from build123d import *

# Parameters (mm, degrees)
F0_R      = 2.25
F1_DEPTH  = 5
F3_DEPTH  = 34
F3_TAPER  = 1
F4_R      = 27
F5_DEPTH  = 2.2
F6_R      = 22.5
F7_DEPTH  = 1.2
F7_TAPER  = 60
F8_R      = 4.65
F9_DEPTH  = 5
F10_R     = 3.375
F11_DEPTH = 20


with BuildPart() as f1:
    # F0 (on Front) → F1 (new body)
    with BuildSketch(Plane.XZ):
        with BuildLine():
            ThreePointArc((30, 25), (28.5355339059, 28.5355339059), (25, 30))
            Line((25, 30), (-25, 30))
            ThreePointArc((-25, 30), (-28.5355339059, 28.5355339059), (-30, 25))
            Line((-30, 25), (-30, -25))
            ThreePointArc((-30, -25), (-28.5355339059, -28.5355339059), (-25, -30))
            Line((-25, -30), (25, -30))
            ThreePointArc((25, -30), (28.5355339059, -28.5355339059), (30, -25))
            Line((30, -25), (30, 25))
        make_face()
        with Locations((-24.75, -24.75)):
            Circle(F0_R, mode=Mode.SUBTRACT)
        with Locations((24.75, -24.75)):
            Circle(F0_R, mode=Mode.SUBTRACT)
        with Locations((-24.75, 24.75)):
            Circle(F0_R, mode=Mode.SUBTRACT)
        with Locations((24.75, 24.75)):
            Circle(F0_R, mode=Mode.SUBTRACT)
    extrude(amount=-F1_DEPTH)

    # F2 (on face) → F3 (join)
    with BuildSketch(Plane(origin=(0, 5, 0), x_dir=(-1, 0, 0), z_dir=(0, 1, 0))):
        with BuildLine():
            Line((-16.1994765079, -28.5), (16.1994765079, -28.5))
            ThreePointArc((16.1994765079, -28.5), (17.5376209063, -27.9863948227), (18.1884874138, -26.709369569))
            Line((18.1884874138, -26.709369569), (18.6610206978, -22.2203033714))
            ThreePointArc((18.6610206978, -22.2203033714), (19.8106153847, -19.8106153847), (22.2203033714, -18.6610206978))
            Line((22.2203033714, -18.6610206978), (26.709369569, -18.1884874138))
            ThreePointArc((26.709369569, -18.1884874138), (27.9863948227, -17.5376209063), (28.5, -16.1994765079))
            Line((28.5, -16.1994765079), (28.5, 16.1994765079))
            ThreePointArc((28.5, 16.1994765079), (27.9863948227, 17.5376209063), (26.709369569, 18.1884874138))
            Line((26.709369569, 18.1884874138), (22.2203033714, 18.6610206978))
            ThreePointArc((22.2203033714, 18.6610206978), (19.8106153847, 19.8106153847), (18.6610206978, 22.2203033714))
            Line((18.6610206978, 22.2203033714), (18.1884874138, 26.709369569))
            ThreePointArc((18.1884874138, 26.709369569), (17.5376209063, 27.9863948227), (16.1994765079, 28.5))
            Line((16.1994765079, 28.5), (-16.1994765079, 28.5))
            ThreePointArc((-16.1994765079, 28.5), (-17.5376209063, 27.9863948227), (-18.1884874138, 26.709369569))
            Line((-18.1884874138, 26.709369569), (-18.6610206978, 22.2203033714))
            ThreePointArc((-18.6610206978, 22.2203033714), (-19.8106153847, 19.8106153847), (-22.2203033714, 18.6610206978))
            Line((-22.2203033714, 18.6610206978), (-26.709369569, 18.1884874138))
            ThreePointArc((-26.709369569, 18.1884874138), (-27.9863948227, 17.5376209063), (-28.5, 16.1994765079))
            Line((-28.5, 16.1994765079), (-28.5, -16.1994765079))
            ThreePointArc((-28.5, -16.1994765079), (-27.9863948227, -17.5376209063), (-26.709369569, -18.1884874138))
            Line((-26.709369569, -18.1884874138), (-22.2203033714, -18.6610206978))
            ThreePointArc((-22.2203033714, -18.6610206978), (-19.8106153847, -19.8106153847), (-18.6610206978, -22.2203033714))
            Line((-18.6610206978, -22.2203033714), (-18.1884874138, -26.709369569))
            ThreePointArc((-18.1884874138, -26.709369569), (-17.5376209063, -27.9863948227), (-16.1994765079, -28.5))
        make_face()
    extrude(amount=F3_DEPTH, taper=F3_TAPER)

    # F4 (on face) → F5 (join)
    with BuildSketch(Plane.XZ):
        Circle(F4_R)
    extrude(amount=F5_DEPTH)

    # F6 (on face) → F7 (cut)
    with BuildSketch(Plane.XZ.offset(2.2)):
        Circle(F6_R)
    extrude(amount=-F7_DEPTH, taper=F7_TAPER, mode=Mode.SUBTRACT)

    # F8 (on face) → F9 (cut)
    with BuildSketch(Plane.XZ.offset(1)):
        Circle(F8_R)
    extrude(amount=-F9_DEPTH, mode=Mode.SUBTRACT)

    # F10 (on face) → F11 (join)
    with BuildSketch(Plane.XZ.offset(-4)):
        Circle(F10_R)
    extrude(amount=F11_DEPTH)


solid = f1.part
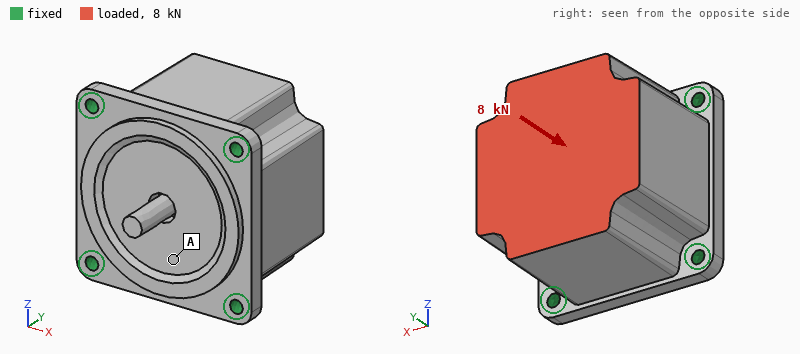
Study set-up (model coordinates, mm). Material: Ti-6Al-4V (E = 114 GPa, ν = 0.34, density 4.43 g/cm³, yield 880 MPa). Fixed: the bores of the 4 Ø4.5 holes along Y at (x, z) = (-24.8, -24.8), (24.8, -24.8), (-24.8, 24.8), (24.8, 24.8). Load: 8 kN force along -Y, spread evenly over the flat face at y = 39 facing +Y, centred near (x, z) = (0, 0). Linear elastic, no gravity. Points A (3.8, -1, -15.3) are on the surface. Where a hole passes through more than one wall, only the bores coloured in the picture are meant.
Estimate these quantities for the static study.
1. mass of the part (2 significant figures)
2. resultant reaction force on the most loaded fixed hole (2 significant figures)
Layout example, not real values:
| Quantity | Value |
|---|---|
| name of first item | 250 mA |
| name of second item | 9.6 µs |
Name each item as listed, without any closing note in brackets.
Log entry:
| Quantity | Value |
|---|---|
| mass of the part | 510 g |
| resultant reaction force on the most loaded fixed hole | 2.1 kN |
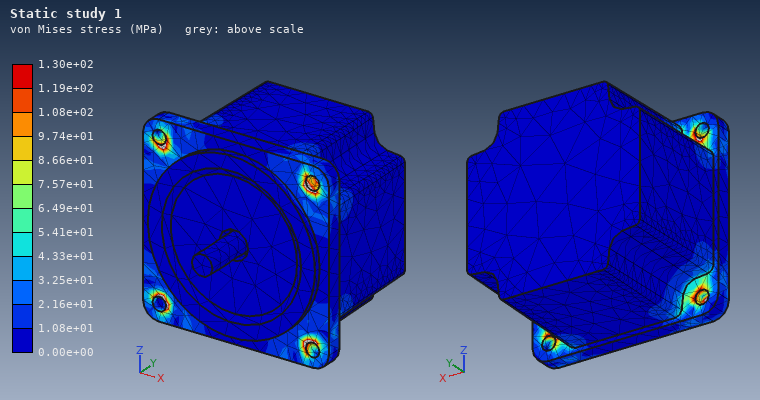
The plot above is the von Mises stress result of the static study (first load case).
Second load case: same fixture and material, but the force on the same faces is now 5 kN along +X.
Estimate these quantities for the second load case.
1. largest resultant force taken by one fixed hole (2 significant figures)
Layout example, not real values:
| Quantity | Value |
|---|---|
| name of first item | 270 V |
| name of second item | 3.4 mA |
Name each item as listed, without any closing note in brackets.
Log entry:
| Quantity | Value |
|---|---|
| largest resultant force taken by one fixed hole | 2.4 kN |
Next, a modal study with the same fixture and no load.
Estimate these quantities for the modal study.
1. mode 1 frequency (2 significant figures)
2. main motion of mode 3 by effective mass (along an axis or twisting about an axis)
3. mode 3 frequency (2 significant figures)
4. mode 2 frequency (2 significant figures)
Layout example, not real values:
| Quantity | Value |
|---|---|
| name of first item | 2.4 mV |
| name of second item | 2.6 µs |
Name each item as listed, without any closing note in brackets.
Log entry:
| Quantity | Value |
|---|---|
| mode 1 frequency | 6100 Hz |
| main motion of mode 3 by effective mass | along Y |
| mode 3 frequency | 7000 Hz |
| mode 2 frequency | 6100 Hz |
